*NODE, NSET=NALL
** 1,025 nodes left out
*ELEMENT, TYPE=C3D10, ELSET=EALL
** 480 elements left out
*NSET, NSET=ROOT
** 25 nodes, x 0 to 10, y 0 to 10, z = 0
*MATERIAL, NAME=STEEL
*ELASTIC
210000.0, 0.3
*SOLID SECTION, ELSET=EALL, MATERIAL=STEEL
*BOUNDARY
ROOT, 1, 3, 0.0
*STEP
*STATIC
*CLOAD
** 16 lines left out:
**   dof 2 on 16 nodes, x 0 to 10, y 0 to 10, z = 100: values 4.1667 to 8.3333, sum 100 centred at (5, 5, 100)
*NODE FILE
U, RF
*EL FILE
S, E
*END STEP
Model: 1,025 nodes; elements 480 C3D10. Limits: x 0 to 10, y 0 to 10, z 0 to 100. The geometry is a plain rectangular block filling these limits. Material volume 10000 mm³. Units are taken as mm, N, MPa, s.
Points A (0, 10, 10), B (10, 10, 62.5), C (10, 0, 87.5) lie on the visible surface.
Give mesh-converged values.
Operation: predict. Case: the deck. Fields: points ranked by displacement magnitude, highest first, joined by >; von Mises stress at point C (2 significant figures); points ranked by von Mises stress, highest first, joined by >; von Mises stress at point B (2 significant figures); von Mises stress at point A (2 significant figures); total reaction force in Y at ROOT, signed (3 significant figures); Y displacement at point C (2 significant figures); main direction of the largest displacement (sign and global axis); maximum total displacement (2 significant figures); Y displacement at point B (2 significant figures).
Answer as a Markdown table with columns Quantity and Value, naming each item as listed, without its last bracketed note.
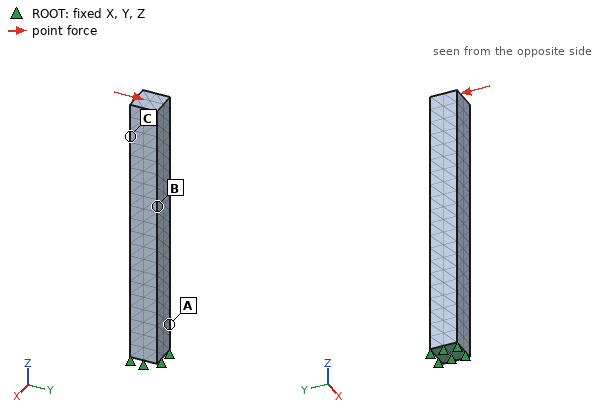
| Quantity | Value |
|---|---|
| points ranked by displacement magnitude, highest first, joined by > | C > B > A |
| von Mises stress at point C | 7.5 MPa |
| points ranked by von Mises stress, highest first, joined by > | A > B > C |
| von Mises stress at point B | 23 MPa |
| von Mises stress at point A | 54 MPa |
| total reaction force in Y at ROOT, signed | -100 N |
| Y displacement at point C | 0.15 mm |
| main direction of the largest displacement | +Y |
| maximum total displacement | 0.19 mm |
| Y displacement at point B | 0.088 mm |
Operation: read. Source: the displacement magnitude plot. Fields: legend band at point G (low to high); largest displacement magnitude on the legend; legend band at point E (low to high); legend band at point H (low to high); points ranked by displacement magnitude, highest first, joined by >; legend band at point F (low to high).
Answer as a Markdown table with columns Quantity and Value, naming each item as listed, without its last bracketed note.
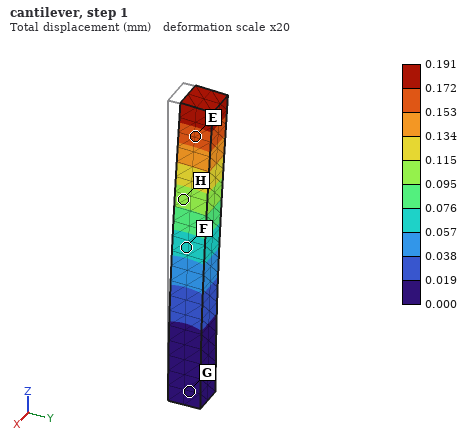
| Quantity | Value |
|---|---|
| legend band at point G | 0.000 to 0.019 mm |
| largest displacement magnitude on the legend | 0.191 mm |
| legend band at point E | 0.153 to 0.172 mm |
| legend band at point H | 0.095 to 0.115 mm |
| points ranked by displacement magnitude, highest first, joined by > | E > H > F > G |
| legend band at point F | 0.057 to 0.076 mm |
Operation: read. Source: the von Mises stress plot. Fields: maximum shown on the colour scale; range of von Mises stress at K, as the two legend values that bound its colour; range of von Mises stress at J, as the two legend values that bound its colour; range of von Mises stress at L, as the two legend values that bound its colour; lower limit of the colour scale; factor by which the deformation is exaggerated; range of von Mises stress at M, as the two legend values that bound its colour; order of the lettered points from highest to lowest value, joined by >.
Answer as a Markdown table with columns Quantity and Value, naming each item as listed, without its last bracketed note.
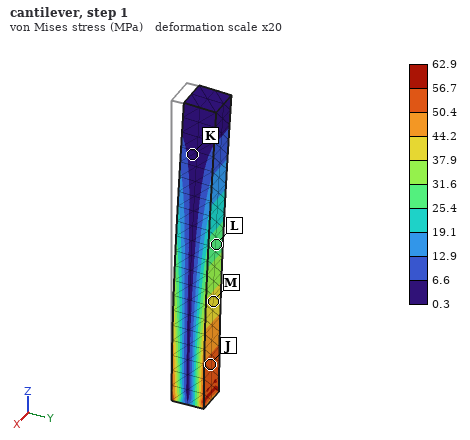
| Quantity | Value |
|---|---|
| maximum shown on the colour scale | 62.9 MPa |
| range of von Mises stress at K, as the two legend values that bound its colour | 0.3 to 6.6 MPa |
| range of von Mises stress at J, as the two legend values that bound its colour | 50.4 to 56.7 MPa |
| range of von Mises stress at L, as the two legend values that bound its colour | 25.4 to 31.6 MPa |
| lower limit of the colour scale | 0.3 MPa |
| factor by which the deformation is exaggerated | 20 |
| range of von Mises stress at M, as the two legend values that bound its colour | 37.9 to 44.2 MPa |
| order of the lettered points from highest to lowest value, joined by > | J > M > L > K |
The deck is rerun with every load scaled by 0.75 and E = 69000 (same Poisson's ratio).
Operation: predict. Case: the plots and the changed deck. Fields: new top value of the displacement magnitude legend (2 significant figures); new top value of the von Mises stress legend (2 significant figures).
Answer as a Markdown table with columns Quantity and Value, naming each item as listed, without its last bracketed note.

| Quantity | Value |
|---|---|
| new top value of the displacement magnitude legend | 0.44 mm |
| new top value of the von Mises stress legend | 47 MPa |
